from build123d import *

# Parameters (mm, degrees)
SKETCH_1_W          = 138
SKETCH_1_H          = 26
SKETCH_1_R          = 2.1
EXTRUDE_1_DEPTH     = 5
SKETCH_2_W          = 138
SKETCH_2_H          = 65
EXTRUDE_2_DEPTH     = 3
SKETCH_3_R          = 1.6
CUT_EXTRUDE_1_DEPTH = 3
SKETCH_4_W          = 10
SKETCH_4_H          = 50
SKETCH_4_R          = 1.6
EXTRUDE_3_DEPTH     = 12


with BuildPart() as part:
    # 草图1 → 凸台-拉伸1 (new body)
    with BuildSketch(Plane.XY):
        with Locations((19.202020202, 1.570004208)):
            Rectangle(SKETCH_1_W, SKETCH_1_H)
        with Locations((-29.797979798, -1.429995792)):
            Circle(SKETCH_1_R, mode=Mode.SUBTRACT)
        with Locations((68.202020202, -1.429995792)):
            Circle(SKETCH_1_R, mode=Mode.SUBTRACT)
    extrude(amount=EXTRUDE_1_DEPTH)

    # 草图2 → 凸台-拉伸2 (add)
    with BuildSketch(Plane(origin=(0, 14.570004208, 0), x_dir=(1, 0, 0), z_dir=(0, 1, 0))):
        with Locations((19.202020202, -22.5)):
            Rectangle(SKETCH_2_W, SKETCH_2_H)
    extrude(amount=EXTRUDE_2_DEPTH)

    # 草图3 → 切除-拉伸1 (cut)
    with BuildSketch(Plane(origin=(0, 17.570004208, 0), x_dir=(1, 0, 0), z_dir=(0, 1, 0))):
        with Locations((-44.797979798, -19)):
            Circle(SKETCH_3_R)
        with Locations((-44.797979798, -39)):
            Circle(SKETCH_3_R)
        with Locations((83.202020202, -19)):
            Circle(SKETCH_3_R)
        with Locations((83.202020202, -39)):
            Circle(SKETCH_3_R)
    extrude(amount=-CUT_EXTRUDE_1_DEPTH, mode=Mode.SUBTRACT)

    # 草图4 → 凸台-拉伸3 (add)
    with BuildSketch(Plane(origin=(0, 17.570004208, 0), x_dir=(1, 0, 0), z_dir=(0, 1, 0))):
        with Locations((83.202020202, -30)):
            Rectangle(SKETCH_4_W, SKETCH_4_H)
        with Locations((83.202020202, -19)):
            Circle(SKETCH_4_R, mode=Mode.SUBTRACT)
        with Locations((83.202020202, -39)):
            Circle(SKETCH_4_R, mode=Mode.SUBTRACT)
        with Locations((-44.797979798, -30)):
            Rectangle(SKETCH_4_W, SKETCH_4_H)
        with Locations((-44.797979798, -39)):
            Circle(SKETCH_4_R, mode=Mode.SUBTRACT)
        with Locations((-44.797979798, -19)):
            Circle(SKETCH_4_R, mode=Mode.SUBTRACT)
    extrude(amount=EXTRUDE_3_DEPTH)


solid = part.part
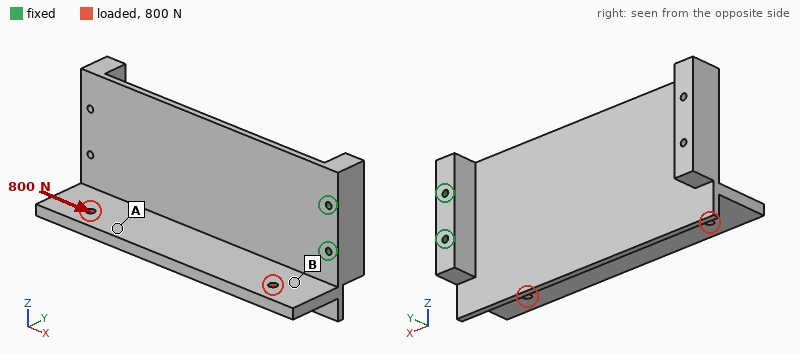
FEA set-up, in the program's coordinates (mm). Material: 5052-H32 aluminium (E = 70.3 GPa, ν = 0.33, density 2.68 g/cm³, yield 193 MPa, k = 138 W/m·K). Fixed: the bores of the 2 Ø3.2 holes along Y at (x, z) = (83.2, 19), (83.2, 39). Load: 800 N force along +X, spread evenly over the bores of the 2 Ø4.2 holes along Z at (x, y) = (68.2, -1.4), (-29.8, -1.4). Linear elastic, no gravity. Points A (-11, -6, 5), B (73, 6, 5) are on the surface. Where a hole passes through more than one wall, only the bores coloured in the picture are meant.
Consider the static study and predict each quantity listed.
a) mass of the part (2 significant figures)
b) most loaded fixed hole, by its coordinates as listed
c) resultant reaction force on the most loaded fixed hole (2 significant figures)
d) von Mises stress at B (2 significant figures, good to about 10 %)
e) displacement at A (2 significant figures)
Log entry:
150 g
(83.2, 19)
1.3 kN
18 MPa
0.64 mm
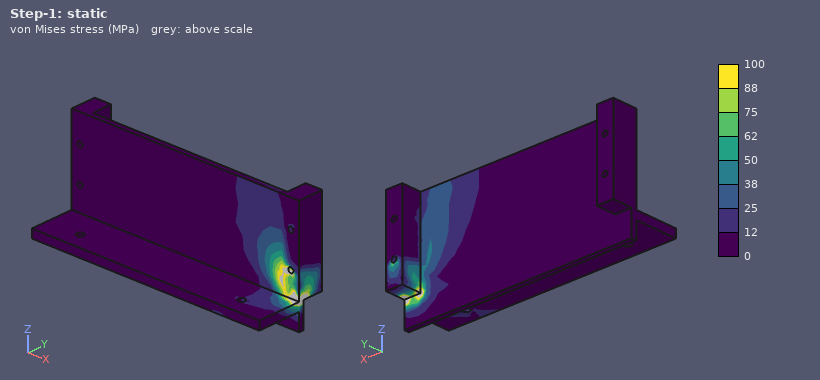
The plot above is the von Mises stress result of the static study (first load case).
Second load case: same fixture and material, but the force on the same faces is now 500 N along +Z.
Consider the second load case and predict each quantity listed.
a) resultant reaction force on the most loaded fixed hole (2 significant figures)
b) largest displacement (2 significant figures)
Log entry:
1.4 kN
0.57 mm
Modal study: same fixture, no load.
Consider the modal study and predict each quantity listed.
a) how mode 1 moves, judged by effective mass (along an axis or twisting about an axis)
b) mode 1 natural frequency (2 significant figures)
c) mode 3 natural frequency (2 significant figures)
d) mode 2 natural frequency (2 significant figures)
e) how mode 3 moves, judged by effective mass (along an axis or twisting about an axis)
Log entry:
along Y
250 Hz
1100 Hz
560 Hz
along Z
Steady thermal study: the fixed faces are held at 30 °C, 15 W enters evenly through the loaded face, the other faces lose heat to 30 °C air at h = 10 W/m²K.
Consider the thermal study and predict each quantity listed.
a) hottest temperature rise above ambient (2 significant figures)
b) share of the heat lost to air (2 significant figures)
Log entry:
25 K
26 %
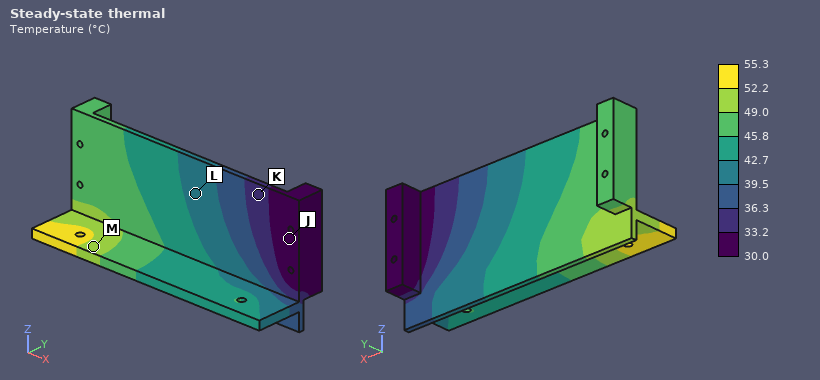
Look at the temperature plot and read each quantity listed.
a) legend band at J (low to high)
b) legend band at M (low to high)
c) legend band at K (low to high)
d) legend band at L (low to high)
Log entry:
30.0 to 33.2 °C
49.0 to 52.2 °C
33.2 to 36.3 °C
39.5 to 42.7 °C
